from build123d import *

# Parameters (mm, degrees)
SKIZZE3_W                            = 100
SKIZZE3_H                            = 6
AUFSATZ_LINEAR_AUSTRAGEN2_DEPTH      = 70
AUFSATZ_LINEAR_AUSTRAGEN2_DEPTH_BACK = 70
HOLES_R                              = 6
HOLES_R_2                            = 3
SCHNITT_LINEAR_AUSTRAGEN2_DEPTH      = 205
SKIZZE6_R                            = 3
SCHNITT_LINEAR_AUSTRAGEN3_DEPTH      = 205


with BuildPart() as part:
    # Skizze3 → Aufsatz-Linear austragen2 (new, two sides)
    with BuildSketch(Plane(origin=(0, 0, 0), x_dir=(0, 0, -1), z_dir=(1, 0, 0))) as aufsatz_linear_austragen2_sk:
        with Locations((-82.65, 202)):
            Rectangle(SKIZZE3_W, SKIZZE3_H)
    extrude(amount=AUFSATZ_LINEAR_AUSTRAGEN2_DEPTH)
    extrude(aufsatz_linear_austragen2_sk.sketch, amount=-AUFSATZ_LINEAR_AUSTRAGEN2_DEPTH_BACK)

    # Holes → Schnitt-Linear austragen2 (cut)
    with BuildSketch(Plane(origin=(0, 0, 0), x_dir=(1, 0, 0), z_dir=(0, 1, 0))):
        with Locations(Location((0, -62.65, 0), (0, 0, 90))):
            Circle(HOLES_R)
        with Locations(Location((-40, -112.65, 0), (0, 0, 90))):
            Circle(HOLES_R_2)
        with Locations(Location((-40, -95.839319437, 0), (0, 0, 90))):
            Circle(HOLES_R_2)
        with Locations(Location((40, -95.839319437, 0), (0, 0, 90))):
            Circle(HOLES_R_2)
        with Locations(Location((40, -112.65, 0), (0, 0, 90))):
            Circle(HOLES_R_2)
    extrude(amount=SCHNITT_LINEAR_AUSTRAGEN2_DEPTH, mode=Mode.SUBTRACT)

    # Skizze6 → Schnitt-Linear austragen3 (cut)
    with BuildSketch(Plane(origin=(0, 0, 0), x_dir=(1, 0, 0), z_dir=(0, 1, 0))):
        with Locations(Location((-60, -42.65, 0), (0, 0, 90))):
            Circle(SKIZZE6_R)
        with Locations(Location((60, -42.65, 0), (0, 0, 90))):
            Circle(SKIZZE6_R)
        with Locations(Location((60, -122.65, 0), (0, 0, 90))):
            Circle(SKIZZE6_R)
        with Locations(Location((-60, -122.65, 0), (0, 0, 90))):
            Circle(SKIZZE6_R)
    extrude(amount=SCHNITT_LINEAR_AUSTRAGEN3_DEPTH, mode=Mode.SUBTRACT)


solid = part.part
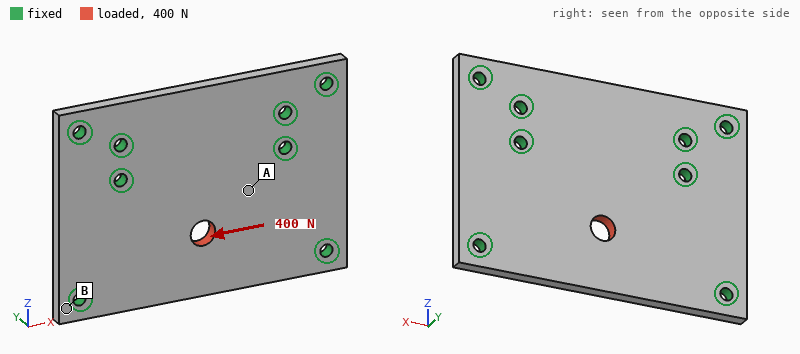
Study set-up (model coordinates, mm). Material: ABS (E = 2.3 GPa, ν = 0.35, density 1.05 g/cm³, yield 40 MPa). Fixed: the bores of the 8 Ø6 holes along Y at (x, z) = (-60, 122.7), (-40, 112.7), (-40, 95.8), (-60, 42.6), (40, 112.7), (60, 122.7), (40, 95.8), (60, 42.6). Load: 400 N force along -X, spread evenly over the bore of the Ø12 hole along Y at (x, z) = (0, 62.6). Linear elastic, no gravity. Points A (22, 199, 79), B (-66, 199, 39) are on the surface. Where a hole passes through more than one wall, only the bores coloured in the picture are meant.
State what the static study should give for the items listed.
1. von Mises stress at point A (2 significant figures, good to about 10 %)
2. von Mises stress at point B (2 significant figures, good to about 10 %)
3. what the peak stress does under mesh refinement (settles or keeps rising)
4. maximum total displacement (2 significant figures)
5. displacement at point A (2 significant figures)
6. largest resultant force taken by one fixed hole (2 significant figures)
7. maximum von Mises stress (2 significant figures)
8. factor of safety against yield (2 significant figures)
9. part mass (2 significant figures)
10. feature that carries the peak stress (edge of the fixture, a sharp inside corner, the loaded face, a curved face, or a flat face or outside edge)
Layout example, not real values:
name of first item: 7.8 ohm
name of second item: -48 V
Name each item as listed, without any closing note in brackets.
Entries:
von Mises stress at point A: 0.69 MPa
von Mises stress at point B: 0.32 MPa
what the peak stress does under mesh refinement: settles
maximum total displacement: 23 µm
displacement at point A: 8.2 µm
largest resultant force taken by one fixed hole: 100 N
maximum von Mises stress: 3.1 MPa
factor of safety against yield: 13
part mass: 86 g
feature that carries the peak stress: the loaded face
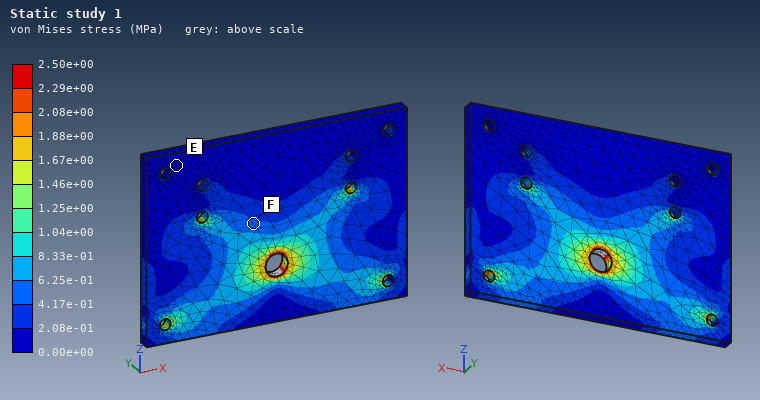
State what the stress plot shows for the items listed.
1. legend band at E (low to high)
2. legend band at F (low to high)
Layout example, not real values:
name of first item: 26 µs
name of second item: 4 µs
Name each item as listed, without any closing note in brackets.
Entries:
legend band at E: 0.00e+00 to 2.08e-01 MPa
legend band at F: 4.17e-01 to 6.25e-01 MPa
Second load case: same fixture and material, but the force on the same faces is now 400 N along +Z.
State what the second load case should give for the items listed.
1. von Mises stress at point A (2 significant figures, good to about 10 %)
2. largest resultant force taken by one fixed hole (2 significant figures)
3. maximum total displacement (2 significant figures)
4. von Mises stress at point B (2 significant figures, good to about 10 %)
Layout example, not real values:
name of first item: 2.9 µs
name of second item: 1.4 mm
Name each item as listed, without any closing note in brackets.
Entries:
von Mises stress at point A: 0.94 MPa
largest resultant force taken by one fixed hole: 110 N
maximum total displacement: 34 µm
von Mises stress at point B: 0.22 MPa
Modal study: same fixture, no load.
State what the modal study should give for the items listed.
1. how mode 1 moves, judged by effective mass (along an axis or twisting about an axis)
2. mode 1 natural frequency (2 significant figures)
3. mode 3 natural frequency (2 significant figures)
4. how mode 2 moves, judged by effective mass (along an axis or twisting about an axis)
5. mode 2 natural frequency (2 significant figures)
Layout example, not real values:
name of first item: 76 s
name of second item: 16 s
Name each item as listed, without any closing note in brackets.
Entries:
how mode 1 moves, judged by effective mass: along Y
mode 1 natural frequency: 760 Hz
mode 3 natural frequency: 1800 Hz
how mode 2 moves, judged by effective mass: along Y
mode 2 natural frequency: 1400 Hz
